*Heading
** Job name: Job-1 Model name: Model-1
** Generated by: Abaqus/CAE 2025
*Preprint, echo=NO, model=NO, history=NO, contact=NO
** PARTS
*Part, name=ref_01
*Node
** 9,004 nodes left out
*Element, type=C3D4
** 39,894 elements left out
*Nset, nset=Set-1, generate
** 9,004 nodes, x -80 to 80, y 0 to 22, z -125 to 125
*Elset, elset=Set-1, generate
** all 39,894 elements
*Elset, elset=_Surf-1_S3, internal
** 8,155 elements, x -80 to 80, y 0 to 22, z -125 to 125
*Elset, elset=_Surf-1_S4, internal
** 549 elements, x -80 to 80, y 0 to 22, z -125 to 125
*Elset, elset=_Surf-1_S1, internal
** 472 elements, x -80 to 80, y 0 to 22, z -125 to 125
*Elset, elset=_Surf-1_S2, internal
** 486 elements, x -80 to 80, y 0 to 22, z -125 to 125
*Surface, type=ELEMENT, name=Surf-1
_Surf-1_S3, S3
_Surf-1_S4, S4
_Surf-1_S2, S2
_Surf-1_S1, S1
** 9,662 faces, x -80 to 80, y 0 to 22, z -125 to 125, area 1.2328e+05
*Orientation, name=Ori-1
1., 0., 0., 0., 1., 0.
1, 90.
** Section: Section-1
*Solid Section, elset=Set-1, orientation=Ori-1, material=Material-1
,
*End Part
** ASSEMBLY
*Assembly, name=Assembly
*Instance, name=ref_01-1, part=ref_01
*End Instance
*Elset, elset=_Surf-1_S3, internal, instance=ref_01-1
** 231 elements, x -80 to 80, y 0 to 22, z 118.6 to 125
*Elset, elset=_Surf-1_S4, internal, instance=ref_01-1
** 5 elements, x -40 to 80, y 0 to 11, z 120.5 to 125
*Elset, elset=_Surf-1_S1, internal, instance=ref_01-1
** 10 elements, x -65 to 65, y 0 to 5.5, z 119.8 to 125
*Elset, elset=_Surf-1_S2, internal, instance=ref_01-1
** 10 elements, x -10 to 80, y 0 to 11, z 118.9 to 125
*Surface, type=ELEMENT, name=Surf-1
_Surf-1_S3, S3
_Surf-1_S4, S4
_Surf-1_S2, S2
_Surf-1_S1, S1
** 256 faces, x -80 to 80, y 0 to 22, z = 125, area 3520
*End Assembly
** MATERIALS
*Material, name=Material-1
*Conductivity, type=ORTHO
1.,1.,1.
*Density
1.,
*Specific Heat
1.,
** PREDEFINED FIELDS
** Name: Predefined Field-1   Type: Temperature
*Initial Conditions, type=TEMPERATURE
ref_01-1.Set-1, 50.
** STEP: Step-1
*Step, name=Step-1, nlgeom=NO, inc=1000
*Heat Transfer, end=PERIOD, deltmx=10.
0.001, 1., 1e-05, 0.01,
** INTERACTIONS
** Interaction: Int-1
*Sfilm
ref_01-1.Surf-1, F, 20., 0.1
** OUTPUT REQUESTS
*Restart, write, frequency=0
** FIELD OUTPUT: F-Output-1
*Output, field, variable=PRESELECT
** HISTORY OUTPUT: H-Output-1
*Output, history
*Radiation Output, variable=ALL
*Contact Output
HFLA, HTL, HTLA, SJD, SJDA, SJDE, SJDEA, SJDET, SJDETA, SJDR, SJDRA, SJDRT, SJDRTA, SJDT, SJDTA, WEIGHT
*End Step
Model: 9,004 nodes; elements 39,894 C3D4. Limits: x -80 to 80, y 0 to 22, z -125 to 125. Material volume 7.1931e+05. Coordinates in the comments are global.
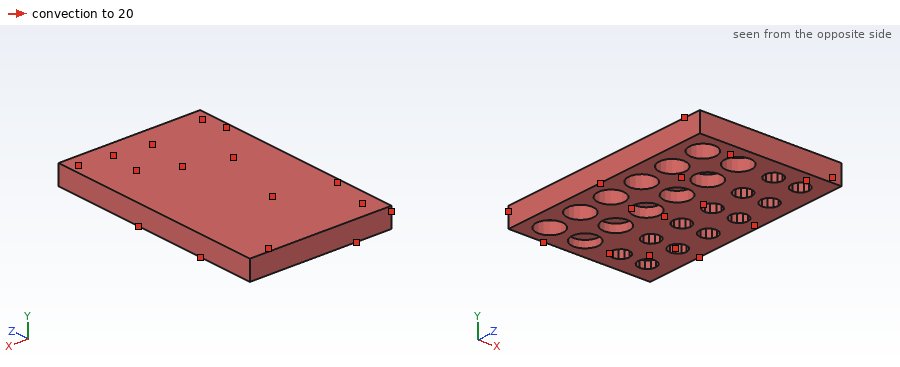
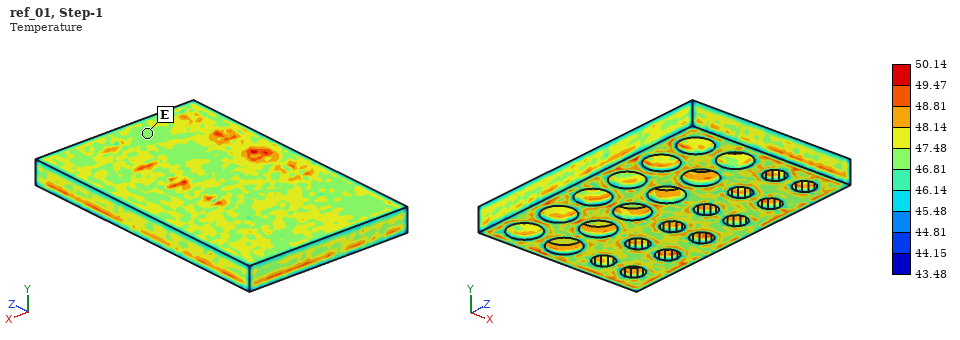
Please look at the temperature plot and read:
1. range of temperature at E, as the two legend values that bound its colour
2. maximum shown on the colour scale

46.81 to 47.48
50.14
